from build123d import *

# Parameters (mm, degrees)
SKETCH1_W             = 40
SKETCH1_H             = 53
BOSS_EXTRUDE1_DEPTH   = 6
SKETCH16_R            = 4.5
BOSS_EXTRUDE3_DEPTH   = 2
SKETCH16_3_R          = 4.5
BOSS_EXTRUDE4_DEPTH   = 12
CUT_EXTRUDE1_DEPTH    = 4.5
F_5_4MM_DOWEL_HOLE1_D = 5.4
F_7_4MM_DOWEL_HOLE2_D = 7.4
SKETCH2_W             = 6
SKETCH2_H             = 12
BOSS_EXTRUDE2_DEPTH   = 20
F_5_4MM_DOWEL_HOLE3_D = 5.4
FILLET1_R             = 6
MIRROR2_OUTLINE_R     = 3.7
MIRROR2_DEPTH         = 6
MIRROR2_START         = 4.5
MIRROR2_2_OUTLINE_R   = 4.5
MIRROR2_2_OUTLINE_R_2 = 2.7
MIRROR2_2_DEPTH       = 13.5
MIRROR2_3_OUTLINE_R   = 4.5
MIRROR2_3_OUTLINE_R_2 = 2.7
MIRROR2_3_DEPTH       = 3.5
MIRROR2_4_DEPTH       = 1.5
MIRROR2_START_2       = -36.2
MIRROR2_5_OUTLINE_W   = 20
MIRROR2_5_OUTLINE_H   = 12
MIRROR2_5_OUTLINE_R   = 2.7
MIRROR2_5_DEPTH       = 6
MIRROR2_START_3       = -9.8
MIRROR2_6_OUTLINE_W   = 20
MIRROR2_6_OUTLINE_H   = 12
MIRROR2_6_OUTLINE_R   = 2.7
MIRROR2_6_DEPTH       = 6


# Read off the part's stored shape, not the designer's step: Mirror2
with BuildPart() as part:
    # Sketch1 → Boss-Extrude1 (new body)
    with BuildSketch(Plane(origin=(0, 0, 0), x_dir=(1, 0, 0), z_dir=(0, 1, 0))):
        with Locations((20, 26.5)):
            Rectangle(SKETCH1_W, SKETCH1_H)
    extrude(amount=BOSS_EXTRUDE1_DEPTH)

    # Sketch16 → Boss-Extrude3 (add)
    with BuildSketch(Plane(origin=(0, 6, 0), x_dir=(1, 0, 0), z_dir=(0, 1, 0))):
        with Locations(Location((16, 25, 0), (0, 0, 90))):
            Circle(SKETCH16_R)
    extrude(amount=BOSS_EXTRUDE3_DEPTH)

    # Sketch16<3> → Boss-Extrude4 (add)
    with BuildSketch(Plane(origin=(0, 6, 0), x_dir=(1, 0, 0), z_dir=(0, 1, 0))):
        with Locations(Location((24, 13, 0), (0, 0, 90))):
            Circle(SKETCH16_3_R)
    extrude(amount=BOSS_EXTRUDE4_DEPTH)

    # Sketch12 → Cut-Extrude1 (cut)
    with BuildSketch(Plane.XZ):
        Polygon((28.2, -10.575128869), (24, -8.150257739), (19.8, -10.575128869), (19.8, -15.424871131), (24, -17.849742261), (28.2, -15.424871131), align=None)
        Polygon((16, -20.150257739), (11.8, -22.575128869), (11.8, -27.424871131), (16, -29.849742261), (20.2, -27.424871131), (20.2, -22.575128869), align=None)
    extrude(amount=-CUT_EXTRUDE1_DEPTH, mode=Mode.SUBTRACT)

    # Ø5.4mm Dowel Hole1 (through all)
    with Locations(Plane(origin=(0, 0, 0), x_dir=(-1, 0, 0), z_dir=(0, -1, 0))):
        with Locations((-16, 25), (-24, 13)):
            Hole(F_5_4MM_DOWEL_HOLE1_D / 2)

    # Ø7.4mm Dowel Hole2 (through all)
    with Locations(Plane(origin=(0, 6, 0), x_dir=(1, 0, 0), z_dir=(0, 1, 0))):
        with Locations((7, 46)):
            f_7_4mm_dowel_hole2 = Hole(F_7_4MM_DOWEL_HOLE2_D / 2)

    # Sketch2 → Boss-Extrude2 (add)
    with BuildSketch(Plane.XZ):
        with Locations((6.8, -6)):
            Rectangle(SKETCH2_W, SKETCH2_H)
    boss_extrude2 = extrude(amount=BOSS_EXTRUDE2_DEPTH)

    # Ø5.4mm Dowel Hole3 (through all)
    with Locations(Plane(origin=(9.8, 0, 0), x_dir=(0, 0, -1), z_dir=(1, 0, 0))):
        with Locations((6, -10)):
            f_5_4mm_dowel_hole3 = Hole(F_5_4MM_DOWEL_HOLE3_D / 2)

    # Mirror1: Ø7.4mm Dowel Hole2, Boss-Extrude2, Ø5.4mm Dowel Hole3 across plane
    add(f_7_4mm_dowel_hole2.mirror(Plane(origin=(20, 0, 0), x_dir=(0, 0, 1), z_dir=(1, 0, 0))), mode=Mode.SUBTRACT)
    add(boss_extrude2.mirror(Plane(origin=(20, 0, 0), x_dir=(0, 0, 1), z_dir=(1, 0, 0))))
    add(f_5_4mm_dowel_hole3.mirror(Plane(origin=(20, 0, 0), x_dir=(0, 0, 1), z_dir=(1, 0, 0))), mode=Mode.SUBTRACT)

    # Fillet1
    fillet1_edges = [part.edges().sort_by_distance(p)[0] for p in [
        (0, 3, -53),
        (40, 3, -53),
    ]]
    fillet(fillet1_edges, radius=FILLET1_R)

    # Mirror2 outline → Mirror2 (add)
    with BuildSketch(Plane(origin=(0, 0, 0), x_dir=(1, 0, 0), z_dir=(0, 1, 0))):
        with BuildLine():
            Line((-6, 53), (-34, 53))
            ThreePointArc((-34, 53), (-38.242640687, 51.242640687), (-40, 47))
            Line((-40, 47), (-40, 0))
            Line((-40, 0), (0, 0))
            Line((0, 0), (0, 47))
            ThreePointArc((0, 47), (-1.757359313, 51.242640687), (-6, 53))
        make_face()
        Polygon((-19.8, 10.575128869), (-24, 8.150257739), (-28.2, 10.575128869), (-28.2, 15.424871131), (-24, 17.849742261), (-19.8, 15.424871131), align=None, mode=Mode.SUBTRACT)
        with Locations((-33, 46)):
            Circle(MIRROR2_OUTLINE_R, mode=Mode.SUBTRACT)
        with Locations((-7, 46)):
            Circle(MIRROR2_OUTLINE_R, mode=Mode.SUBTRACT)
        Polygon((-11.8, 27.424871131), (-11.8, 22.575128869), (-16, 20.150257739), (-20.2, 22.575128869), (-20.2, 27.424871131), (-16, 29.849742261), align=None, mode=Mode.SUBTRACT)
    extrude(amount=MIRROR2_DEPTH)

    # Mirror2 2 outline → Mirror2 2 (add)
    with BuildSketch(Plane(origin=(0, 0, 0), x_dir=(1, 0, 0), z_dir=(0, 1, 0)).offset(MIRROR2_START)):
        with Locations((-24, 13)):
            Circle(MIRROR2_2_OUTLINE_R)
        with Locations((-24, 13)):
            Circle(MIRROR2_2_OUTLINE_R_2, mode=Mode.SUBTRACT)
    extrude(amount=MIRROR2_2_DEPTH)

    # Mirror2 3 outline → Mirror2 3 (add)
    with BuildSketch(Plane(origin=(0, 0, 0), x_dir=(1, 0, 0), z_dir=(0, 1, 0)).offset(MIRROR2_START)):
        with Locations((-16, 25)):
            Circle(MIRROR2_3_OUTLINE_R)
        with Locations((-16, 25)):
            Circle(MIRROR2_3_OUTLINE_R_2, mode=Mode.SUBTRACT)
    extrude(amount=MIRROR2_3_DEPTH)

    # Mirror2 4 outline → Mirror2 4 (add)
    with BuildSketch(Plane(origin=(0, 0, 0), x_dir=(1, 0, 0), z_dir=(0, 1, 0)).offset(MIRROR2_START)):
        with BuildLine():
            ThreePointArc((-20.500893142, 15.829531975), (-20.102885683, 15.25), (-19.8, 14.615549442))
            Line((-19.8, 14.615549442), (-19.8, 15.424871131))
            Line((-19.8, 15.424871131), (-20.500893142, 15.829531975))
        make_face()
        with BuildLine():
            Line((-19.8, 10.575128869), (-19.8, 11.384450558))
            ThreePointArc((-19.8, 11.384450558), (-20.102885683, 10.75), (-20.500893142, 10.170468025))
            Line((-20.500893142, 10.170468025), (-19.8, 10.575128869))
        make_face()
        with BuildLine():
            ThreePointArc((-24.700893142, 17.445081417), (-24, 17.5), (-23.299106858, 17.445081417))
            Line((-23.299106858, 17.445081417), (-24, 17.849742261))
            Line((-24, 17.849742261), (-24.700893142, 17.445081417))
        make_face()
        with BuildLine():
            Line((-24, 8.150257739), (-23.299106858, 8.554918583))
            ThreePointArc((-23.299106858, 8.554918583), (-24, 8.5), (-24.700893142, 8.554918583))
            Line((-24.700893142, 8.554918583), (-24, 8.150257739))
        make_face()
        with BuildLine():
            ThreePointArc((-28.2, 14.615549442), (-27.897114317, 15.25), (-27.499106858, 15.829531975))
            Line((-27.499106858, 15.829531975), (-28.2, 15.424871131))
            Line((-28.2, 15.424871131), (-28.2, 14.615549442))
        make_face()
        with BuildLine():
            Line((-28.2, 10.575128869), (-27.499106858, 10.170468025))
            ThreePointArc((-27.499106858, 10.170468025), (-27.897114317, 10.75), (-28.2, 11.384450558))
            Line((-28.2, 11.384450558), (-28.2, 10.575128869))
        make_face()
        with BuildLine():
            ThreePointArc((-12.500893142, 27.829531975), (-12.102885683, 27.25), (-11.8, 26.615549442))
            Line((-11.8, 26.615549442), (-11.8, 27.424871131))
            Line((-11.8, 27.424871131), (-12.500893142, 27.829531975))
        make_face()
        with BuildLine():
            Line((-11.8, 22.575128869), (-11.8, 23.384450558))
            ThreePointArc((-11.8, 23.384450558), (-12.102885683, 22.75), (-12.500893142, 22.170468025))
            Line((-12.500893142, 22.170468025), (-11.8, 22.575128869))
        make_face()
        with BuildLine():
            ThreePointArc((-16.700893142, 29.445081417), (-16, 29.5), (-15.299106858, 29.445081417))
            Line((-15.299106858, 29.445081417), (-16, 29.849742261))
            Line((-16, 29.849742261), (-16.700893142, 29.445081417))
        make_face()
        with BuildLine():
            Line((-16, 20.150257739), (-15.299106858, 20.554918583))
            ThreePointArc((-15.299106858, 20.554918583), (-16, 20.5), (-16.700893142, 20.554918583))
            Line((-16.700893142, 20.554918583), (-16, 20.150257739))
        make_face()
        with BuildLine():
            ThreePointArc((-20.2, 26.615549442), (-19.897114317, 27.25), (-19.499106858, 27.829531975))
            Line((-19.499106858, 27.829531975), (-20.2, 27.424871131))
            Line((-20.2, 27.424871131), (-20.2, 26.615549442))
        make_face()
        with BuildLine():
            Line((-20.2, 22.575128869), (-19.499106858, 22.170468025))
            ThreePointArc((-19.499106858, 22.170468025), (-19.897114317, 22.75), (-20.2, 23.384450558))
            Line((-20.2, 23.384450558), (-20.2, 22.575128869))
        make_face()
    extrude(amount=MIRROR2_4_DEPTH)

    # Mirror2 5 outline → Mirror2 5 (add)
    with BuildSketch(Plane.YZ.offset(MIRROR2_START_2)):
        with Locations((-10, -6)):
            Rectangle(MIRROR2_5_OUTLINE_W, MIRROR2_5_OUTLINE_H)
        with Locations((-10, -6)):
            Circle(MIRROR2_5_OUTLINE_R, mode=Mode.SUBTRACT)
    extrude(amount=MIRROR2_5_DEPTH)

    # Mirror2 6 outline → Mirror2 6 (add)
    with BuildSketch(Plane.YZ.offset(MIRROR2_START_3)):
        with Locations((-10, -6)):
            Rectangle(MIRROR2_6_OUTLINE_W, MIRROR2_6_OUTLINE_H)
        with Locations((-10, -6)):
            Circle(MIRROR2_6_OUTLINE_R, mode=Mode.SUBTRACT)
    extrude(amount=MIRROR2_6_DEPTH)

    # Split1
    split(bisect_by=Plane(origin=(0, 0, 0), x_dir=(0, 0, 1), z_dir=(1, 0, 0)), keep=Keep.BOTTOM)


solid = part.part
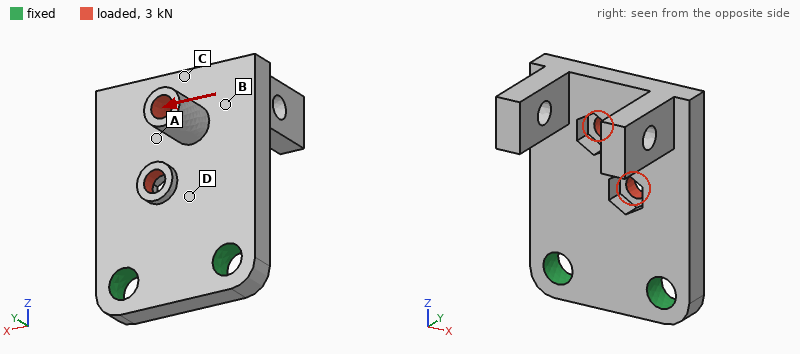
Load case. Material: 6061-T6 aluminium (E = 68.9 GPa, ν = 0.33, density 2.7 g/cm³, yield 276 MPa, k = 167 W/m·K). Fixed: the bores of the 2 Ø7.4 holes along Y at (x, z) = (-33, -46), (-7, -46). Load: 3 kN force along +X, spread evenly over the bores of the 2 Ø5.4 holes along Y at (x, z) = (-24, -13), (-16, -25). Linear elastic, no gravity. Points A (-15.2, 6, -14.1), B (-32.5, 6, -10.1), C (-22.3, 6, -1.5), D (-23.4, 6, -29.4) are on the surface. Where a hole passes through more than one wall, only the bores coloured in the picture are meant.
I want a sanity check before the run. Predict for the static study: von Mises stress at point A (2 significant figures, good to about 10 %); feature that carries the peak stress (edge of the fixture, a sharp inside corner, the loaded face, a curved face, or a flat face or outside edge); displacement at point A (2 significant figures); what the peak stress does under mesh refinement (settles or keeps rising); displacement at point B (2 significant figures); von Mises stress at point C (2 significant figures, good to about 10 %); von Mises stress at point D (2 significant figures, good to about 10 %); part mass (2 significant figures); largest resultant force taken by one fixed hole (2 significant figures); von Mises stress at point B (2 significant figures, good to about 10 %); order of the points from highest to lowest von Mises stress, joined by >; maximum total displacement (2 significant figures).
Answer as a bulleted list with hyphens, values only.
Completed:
- 70 MPa
- a sharp inside corner
- 0.059 mm
- keeps rising
- 0.091 mm
- 30 MPa
- 95 MPa
- 40 g
- 3.4 kN
- 56 MPa
- D > A > B > C
- 0.22 mm
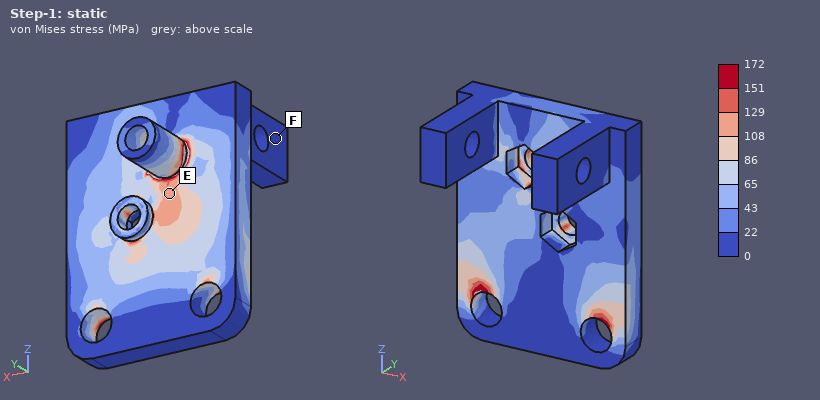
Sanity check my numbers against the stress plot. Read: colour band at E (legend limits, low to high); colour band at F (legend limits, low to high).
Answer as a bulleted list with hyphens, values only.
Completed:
- 108 to 129 MPa
- 0 to 22 MPa
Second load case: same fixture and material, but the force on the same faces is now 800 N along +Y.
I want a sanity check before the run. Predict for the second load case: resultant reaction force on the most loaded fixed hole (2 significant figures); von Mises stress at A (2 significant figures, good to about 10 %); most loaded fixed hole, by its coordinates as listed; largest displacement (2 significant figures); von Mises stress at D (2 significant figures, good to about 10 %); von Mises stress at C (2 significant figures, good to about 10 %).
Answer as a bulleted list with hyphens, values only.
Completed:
- 460 N
- 15 MPa
- (-33, -46)
- 0.31 mm
- 51 MPa
- 19 MPa
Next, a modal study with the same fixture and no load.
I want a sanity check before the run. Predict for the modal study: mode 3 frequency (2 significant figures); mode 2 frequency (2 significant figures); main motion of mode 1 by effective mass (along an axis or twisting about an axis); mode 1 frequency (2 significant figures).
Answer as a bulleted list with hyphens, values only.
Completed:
- 6400 Hz
- 3600 Hz
- along Y
- 1800 Hz
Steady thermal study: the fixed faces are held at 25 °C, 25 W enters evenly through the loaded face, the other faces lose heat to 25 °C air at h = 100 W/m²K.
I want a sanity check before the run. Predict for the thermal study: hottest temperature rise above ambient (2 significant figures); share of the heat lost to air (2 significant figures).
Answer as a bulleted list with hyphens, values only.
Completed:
- 35 K
- 29 %
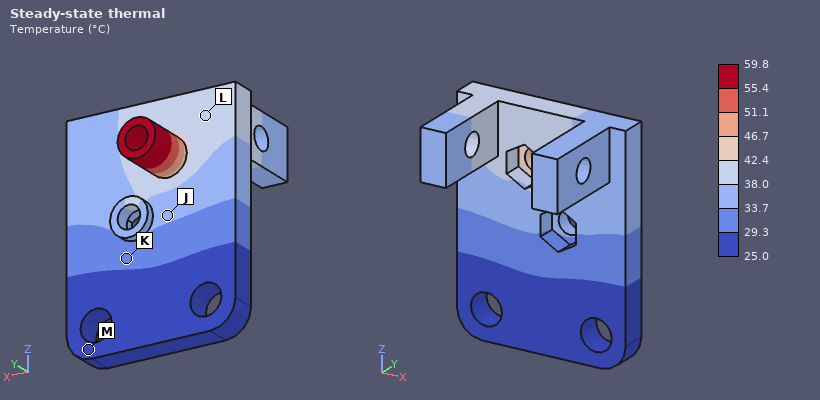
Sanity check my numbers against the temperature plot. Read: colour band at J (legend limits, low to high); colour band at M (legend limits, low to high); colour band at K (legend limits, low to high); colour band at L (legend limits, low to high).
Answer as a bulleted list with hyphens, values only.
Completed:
- 33.7 to 38.0 °C
- 25.0 to 29.3 °C
- 29.3 to 33.7 °C
- 38.0 to 42.4 °C
